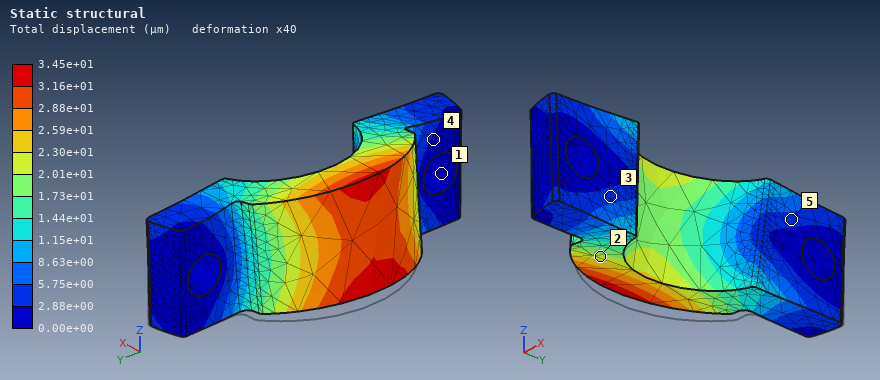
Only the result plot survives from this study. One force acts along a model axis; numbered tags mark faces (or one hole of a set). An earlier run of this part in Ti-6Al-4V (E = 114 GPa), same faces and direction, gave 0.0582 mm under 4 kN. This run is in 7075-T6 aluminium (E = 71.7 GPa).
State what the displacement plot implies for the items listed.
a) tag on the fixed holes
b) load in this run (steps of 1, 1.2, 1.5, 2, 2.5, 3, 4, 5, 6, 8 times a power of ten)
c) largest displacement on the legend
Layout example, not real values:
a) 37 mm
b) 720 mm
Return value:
a) 1
b) 1.5 kN
c) 3.45e+01 µm
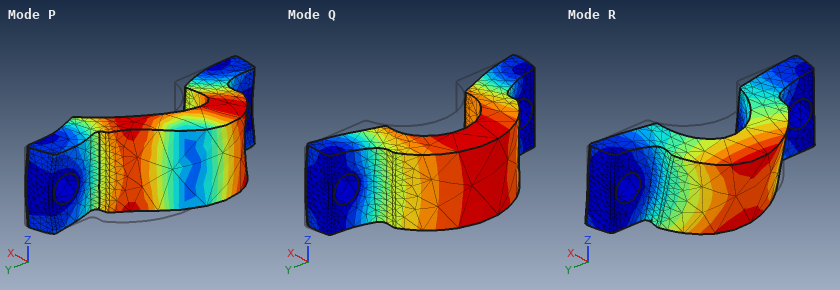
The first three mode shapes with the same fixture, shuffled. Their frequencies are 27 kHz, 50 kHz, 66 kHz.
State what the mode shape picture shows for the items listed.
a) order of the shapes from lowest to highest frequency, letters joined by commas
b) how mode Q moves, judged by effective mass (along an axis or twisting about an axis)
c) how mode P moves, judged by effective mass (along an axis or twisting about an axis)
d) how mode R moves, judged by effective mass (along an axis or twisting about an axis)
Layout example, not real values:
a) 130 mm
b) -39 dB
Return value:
a) R, Q, P
b) along X
c) along Y
d) along Z
